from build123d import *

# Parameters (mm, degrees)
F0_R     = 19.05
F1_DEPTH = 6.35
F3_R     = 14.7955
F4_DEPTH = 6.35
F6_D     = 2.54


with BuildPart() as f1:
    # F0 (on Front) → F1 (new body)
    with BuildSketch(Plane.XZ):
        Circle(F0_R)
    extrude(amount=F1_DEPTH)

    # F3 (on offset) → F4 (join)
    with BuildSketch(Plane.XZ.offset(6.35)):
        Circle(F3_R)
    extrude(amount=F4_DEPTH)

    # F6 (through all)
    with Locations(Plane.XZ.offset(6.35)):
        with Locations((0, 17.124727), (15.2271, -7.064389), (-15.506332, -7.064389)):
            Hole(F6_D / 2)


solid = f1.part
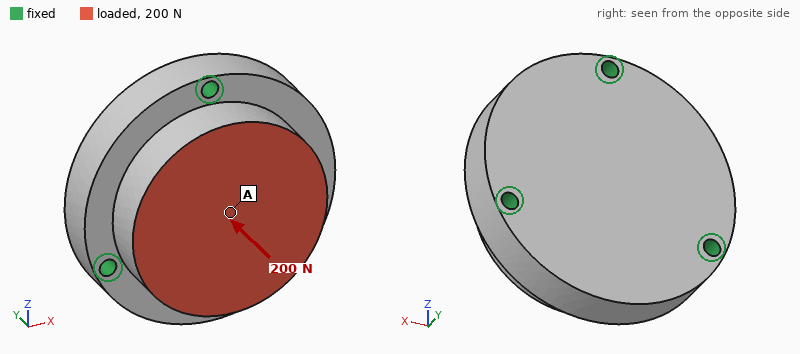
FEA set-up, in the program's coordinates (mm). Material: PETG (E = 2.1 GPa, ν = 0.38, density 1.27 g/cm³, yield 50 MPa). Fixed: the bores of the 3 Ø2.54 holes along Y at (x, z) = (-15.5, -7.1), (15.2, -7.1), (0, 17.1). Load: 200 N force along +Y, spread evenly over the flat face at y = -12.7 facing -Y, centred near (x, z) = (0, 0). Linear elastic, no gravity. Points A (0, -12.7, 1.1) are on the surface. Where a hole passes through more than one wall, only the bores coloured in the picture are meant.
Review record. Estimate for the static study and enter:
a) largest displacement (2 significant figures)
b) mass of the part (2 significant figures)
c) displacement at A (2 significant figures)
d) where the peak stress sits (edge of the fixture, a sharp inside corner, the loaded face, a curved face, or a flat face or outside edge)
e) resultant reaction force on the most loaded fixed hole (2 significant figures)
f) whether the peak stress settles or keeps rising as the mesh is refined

15 µm
15 g
12 µm
edge of the fixture
75 N
keeps rising
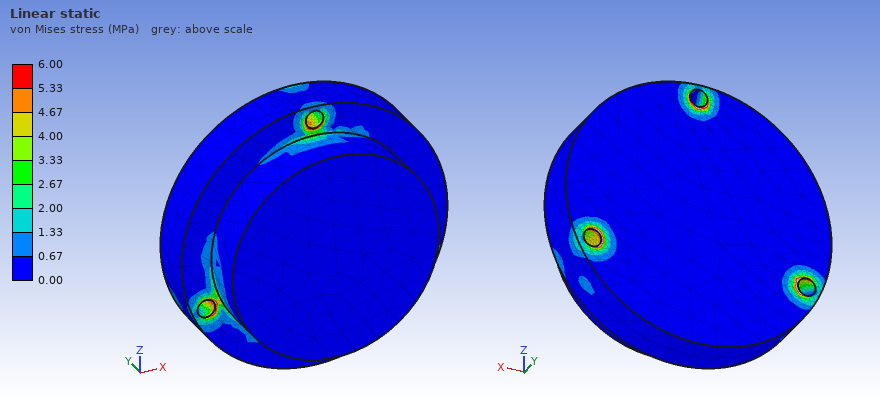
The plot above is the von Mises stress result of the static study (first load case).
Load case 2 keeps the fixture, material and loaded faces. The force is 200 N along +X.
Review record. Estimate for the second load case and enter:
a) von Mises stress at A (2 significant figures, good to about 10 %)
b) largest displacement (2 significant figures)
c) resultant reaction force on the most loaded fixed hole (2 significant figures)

0.79 MPa
18 µm
99 N
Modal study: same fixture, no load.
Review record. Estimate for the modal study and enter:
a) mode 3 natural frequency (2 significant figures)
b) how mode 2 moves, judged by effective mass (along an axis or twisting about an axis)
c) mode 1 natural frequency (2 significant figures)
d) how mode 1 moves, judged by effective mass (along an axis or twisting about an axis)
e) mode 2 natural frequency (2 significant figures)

6900 Hz
along Y
5600 Hz
along Y
6300 Hz
